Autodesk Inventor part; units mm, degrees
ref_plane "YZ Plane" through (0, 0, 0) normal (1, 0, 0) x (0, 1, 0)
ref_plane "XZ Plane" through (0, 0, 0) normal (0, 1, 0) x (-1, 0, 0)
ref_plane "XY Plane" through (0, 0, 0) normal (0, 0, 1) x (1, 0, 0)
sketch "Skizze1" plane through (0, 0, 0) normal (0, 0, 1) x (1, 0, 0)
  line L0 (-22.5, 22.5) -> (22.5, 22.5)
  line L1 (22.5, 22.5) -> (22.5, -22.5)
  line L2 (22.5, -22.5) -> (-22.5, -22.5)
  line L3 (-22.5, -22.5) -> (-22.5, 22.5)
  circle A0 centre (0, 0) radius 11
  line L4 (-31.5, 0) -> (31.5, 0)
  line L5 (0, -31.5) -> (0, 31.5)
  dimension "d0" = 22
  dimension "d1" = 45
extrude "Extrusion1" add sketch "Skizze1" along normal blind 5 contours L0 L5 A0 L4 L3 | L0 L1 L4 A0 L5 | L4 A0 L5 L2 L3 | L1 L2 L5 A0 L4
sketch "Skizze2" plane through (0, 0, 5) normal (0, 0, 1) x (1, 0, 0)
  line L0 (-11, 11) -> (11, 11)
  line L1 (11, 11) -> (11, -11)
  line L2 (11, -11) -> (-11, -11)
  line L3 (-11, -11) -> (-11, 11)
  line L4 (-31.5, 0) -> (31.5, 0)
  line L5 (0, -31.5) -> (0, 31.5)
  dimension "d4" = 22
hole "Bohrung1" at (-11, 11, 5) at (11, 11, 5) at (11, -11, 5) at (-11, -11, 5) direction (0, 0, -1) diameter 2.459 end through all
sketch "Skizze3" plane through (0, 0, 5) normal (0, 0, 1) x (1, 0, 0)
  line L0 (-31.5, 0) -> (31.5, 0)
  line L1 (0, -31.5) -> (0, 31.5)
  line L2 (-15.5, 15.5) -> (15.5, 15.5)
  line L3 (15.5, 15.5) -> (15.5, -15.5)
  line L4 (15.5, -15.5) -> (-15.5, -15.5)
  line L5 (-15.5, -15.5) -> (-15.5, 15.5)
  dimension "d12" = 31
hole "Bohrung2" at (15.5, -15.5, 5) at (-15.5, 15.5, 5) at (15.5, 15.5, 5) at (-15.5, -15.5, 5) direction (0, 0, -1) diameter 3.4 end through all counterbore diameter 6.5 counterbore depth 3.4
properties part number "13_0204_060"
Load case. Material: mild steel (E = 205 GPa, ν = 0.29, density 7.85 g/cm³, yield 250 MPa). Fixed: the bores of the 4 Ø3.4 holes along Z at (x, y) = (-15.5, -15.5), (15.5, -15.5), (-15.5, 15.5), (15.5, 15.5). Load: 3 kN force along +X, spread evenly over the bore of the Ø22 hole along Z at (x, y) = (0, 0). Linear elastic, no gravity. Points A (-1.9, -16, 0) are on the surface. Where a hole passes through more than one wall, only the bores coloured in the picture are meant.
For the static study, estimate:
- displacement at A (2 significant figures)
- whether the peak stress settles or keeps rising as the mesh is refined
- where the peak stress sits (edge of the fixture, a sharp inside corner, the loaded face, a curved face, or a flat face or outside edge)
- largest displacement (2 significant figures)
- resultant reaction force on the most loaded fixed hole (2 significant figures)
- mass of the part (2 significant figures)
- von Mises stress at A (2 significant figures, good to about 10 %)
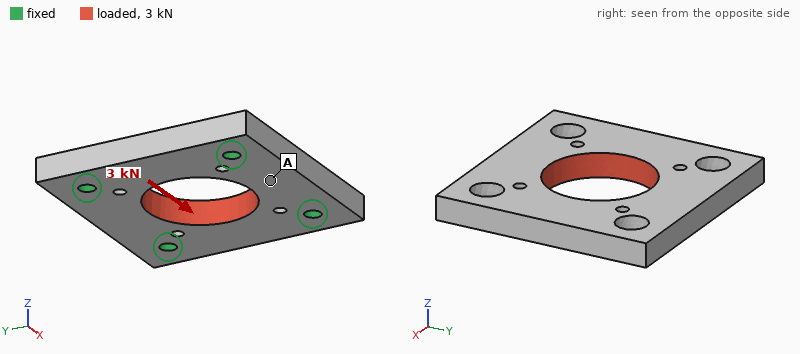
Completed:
1.3 µm
keeps rising
edge of the fixture
2.8 µm
760 N
60 g
14 MPa
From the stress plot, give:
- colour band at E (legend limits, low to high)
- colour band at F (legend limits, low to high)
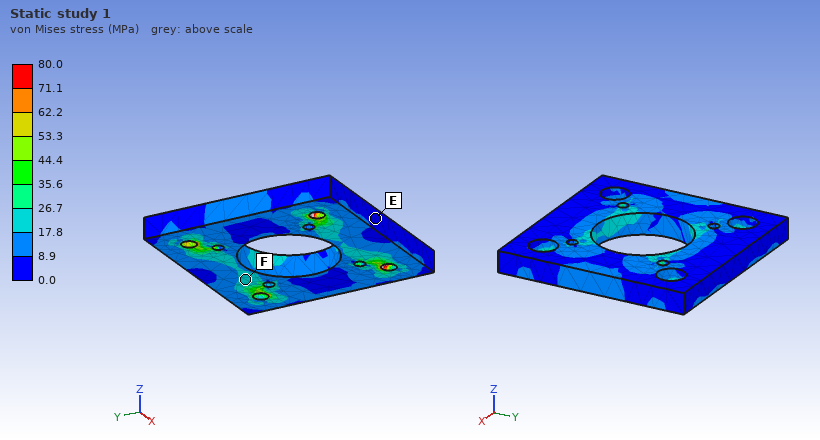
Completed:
0.0 to 8.9 MPa
17.8 to 26.7 MPa
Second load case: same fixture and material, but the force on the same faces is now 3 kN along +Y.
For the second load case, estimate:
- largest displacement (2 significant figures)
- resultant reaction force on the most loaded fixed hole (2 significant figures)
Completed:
2.8 µm
760 N
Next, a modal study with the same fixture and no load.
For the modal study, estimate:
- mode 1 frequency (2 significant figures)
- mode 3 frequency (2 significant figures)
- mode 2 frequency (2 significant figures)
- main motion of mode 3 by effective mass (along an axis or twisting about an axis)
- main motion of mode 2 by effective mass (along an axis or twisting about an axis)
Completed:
15 kHz
18 kHz
16 kHz
twisting about X
along Z
